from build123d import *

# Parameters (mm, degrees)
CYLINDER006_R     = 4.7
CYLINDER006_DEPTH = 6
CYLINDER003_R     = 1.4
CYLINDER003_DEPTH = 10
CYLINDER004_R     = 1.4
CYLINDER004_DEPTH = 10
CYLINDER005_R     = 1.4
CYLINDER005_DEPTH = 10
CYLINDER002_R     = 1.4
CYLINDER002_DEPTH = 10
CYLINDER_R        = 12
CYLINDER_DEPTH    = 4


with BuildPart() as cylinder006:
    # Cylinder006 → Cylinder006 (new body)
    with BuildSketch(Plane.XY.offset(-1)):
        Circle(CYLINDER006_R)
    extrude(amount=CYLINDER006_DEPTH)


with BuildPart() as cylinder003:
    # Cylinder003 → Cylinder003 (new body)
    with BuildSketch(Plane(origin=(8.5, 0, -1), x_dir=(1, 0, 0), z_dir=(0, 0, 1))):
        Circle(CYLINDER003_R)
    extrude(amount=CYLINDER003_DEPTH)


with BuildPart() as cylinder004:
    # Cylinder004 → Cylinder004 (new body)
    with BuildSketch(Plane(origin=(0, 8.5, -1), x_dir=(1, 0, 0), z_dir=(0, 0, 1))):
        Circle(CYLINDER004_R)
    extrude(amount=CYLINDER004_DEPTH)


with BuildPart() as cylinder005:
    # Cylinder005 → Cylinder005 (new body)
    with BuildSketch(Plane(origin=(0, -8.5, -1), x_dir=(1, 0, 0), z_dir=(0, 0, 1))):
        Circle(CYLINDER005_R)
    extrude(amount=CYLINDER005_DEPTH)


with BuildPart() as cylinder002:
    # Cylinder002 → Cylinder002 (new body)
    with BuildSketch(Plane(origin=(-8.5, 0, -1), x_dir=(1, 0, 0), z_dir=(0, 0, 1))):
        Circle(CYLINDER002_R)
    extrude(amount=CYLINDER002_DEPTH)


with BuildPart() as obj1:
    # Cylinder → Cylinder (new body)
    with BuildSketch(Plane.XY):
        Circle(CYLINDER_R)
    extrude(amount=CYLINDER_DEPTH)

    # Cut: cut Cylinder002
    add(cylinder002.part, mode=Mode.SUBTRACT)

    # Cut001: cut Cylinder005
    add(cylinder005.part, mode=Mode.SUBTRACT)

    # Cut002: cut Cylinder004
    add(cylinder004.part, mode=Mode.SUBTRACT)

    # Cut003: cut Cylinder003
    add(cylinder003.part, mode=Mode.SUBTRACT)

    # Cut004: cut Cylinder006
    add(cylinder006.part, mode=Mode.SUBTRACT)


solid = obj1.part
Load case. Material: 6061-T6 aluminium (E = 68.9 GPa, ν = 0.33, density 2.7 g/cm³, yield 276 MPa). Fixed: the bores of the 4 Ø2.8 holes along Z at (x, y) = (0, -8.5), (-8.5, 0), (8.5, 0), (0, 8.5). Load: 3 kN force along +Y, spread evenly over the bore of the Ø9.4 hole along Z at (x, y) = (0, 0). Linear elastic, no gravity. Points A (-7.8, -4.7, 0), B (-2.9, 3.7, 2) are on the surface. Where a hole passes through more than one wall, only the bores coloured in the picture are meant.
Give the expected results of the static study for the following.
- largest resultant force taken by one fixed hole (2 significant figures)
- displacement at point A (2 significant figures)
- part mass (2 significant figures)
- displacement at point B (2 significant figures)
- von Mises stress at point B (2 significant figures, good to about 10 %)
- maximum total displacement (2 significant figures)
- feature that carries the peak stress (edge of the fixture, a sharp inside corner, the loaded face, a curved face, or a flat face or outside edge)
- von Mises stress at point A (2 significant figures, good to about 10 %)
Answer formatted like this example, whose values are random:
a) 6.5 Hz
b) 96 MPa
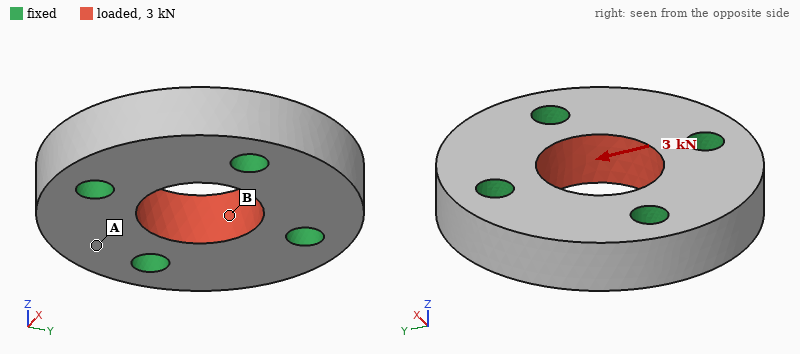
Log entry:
a) 820 N
b) 1.2 µm
c) 3.9 g
d) 2.5 µm
e) 34 MPa
f) 2.8 µm
g) edge of the fixture
h) 13 MPa
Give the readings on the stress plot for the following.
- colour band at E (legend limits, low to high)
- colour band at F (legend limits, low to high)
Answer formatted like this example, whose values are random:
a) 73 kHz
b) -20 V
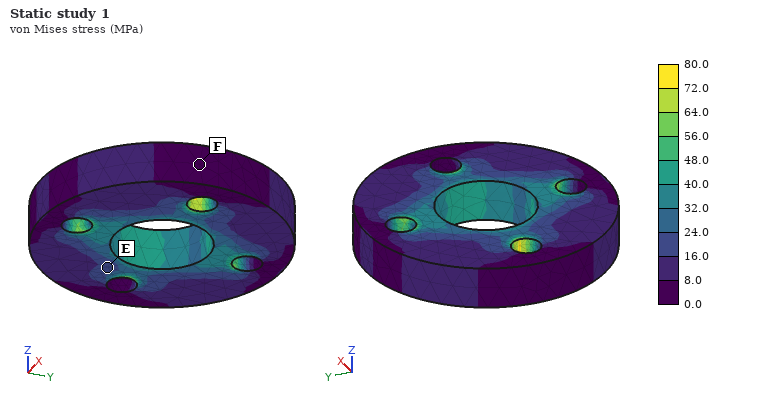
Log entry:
a) 16.0 to 24.0 MPa
b) 0.0 to 8.0 MPa
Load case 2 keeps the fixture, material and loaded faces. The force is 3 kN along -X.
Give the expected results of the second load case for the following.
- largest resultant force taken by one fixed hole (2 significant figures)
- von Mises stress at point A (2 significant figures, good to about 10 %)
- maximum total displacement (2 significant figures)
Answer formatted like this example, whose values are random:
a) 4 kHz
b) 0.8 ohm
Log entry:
a) 820 N
b) 12 MPa
c) 2.8 µm
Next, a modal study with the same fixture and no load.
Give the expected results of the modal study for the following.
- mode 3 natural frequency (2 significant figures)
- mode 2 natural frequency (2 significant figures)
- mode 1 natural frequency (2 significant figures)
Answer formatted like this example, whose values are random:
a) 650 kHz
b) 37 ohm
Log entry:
a) 74 kHz
b) 74 kHz
c) 72 kHz
